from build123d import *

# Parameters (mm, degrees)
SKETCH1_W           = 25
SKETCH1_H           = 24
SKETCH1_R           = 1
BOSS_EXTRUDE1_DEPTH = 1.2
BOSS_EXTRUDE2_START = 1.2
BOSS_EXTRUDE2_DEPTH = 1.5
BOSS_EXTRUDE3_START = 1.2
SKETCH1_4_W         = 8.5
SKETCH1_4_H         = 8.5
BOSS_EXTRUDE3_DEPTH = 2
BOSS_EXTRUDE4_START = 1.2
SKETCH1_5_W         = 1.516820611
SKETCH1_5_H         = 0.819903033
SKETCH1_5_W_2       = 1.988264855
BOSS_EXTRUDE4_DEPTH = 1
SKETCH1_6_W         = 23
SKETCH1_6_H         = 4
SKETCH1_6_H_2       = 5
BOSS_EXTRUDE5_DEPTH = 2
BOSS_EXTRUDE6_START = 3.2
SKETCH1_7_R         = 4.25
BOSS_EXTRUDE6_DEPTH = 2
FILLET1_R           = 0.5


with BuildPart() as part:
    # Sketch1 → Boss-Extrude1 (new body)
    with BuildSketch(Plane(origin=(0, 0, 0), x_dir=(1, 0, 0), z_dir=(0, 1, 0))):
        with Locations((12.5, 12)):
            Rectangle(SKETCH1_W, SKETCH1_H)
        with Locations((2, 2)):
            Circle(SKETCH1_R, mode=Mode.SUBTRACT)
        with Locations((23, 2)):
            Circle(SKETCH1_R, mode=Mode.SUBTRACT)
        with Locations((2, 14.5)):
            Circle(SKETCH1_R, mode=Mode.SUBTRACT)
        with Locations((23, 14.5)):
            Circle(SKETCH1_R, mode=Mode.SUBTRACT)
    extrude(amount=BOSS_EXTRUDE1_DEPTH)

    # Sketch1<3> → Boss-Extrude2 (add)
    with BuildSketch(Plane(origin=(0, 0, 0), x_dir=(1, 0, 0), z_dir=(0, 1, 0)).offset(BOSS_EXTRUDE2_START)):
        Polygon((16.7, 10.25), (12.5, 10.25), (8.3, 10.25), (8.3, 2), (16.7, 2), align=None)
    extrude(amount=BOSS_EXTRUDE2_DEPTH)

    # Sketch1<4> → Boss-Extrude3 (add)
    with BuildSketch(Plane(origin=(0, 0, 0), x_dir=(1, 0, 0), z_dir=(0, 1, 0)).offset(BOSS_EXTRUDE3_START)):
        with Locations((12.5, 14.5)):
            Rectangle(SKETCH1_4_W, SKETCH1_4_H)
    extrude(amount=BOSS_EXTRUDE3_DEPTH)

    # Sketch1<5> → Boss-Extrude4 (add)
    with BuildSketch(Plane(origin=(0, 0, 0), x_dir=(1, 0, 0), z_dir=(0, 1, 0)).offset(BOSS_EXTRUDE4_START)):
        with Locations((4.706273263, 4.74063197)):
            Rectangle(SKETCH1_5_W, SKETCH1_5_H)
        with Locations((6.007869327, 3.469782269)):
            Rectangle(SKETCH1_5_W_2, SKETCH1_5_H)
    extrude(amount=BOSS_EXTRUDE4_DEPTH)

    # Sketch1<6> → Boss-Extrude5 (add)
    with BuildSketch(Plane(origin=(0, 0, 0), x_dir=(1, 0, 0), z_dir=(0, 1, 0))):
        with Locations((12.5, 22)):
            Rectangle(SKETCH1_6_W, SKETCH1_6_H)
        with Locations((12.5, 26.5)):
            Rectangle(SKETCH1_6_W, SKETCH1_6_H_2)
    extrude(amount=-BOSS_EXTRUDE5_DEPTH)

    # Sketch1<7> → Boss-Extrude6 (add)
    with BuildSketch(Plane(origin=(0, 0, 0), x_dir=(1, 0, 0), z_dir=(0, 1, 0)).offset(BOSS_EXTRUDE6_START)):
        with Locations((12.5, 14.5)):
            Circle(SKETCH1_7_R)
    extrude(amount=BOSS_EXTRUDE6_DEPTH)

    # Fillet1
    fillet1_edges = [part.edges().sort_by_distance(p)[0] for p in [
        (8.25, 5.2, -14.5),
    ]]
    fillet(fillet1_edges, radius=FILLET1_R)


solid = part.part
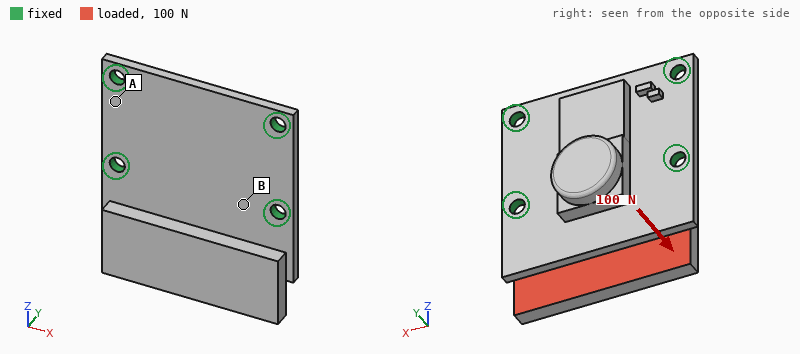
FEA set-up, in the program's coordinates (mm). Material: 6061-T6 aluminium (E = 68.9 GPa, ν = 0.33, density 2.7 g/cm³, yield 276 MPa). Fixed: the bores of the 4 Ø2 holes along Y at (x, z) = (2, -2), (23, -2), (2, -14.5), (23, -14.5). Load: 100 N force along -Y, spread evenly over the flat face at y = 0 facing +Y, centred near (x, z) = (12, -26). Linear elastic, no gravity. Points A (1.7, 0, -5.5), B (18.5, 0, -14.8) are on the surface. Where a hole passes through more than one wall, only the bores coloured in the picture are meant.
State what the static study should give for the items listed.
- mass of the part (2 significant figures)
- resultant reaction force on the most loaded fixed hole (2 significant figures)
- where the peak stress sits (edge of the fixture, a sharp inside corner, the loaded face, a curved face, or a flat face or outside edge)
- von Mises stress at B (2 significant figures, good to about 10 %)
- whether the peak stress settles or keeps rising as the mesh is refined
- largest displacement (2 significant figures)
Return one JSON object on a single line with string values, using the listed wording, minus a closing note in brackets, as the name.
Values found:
{"mass of the part": "4.0 g", "resultant reaction force on the most loaded fixed hole": "93 N", "where the peak stress sits": "edge of the fixture", "von Mises stress at B": "39 MPa", "whether the peak stress settles or keeps rising as the mesh is refined": "keeps rising", "largest displacement": "0.17 mm"}
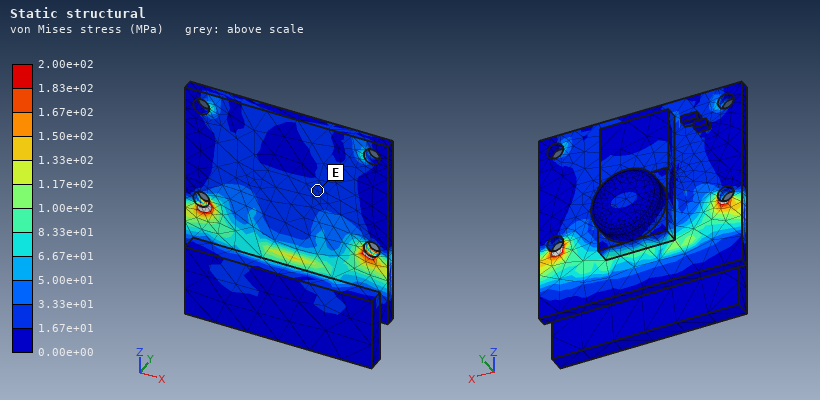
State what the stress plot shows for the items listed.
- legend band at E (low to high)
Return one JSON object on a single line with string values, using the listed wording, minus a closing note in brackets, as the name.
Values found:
{"legend band at E": "1.67e+01 to 3.33e+01 MPa"}
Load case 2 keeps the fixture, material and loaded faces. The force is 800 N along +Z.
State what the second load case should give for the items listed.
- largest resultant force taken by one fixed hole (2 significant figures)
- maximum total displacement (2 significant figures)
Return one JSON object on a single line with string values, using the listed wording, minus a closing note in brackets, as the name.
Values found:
{"largest resultant force taken by one fixed hole": "330 N", "maximum total displacement": "81 µm"}
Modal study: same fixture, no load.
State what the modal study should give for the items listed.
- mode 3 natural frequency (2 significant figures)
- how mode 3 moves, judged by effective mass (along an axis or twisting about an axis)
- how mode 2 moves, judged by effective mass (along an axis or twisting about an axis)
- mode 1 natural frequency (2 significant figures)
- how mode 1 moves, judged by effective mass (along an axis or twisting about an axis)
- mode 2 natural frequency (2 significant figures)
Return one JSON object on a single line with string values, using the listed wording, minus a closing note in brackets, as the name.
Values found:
{"mode 3 natural frequency": "14 kHz", "how mode 3 moves, judged by effective mass": "along Y", "how mode 2 moves, judged by effective mass": "twisting about Z", "mode 1 natural frequency": "4500 Hz", "how mode 1 moves, judged by effective mass": "along Y", "mode 2 natural frequency": "12 kHz"}
